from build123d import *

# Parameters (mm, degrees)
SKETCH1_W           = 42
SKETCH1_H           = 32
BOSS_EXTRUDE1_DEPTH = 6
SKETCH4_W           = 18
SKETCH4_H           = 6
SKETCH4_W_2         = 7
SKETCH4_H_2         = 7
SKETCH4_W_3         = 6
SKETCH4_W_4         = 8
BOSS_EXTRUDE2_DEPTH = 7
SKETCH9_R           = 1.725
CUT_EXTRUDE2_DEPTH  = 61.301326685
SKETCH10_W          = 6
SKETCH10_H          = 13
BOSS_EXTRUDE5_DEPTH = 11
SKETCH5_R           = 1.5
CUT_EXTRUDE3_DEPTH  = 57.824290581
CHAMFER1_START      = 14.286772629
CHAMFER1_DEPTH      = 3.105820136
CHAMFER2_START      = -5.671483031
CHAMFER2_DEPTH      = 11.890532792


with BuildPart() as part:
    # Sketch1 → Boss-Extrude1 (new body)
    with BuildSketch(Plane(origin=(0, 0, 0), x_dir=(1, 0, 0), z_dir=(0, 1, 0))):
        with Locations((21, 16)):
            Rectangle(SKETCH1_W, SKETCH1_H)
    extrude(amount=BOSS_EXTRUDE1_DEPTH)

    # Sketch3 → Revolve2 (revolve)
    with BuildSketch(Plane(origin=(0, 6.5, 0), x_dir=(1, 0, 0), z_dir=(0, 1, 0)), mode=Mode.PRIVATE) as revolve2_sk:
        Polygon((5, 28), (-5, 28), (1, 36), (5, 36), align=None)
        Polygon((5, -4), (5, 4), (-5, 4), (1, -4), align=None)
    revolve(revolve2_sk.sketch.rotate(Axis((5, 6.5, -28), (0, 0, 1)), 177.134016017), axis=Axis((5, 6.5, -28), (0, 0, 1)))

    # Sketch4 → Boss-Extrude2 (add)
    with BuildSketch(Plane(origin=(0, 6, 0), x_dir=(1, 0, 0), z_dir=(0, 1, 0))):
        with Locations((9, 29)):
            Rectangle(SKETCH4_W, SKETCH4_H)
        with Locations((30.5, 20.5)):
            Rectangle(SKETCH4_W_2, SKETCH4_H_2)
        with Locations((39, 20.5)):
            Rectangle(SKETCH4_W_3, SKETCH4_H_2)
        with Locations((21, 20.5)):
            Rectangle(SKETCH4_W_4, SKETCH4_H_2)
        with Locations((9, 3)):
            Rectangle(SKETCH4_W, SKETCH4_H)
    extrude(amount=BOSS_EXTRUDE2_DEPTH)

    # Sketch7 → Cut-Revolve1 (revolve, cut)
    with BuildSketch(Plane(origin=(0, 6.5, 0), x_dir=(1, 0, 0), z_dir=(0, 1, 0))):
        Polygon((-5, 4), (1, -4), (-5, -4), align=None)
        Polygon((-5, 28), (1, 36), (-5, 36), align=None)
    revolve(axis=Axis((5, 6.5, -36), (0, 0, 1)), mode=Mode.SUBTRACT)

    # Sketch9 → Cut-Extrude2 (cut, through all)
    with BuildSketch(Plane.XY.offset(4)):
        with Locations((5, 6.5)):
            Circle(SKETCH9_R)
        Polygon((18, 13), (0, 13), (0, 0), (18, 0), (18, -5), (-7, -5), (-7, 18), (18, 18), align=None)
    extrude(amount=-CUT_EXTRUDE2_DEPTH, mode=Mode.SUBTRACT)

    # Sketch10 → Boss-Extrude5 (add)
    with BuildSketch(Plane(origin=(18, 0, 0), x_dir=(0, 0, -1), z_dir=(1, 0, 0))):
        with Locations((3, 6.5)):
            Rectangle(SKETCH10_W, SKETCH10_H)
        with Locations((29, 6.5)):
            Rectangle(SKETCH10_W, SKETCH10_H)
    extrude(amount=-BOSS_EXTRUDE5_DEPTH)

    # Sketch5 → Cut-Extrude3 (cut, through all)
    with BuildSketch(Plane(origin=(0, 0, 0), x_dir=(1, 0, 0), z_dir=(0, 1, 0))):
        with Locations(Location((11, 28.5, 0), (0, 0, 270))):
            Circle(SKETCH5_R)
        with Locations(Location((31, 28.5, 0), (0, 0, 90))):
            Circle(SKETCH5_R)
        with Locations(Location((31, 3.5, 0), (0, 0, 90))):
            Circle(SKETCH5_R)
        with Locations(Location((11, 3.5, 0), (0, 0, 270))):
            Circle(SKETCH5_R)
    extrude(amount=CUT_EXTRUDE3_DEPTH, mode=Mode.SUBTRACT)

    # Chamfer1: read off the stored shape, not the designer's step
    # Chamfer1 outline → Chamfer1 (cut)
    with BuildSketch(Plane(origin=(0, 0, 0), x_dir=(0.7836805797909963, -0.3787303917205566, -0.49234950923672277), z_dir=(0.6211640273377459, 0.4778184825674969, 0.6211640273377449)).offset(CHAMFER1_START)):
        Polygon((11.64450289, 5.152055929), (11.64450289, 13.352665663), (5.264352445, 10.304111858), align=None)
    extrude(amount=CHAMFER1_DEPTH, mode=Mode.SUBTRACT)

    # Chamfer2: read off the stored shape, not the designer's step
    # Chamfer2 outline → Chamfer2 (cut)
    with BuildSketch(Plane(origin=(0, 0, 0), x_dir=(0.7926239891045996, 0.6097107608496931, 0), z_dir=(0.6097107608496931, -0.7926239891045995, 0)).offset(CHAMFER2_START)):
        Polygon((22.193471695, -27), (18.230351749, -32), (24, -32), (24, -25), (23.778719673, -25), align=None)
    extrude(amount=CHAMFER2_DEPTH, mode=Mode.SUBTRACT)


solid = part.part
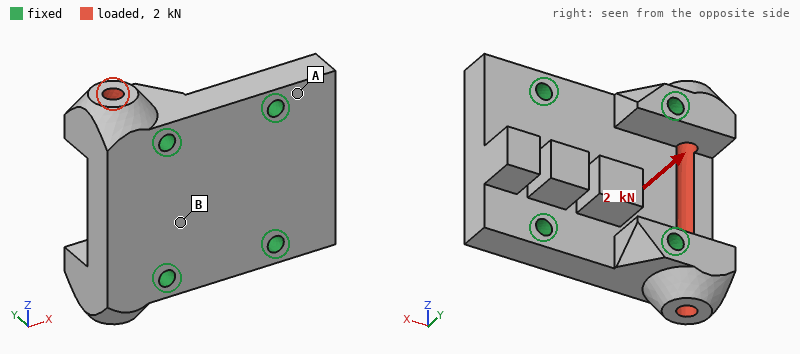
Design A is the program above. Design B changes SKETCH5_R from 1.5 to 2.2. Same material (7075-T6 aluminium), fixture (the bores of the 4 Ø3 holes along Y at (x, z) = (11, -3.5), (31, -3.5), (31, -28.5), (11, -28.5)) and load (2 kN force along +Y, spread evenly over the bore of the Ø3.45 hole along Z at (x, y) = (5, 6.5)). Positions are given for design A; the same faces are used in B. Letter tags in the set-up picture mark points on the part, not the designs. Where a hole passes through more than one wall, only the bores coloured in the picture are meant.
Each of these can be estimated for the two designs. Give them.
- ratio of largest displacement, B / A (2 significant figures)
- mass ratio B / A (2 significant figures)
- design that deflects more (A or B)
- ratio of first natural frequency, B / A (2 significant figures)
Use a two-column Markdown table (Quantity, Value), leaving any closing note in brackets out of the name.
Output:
| Quantity | Value |
|---|---|
| ratio of largest displacement, B / A | 0.85 |
| mass ratio B / A | 0.97 |
| design that deflects more | A |
| ratio of first natural frequency, B / A | 1.1 |
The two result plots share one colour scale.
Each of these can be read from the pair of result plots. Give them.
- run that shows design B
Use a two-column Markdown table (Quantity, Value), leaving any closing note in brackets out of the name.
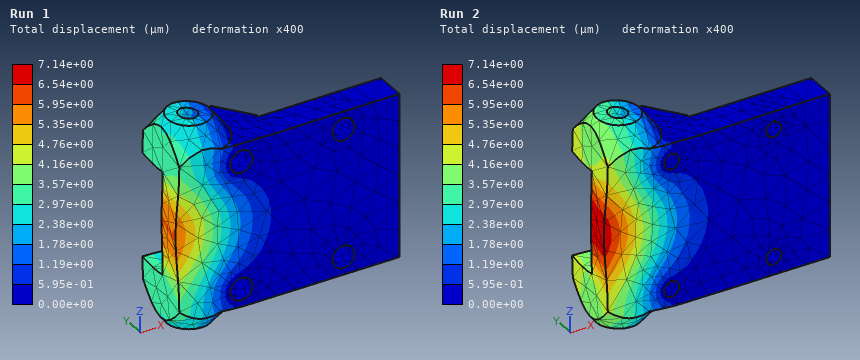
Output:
| Quantity | Value |
|---|---|
| run that shows design B | Run 1 |
